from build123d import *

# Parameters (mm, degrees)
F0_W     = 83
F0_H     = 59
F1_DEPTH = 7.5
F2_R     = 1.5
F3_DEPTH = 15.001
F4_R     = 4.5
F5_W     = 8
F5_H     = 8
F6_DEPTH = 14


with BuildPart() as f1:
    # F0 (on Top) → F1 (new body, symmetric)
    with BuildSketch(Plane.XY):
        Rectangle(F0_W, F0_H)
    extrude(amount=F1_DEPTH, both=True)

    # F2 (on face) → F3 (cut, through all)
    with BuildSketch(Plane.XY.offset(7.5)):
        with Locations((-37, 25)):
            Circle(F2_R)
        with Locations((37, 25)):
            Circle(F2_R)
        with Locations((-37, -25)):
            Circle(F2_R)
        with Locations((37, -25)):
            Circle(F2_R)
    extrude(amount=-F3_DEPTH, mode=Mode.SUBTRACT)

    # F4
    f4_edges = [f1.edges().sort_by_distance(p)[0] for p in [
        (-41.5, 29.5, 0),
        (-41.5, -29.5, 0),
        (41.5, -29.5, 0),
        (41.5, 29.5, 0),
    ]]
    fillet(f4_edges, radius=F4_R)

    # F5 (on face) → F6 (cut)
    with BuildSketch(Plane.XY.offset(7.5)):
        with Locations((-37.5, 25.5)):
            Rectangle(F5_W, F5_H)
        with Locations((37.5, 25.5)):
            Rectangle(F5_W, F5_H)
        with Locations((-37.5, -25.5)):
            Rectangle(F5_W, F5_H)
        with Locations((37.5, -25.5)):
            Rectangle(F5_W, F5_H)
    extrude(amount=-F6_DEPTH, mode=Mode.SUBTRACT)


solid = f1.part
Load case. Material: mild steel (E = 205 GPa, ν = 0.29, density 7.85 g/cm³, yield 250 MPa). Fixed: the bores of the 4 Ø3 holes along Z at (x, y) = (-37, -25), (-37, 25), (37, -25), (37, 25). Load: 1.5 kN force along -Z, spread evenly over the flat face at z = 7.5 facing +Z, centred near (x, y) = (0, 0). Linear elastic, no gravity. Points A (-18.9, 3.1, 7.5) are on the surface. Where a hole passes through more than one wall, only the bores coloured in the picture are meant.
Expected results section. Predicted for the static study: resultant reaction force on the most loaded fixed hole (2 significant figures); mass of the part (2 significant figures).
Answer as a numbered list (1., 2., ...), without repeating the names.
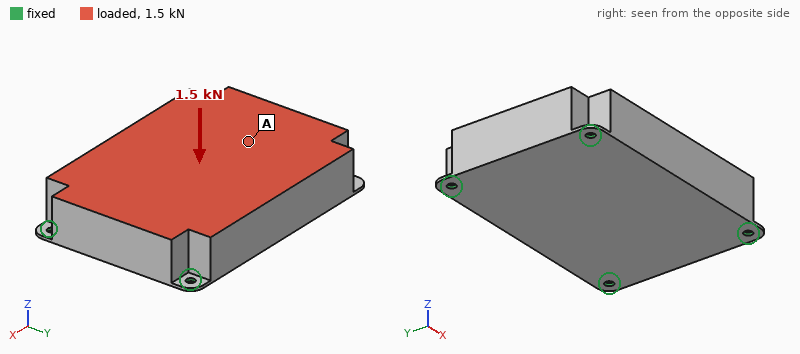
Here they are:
1. 450 N
2. 550 g
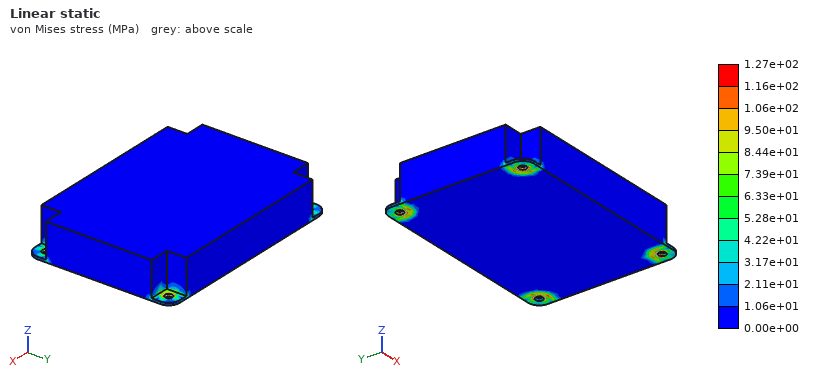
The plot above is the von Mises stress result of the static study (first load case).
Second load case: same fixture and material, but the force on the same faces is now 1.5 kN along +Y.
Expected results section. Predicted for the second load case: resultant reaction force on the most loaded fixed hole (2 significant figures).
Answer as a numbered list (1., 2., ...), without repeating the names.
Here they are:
1. 460 N
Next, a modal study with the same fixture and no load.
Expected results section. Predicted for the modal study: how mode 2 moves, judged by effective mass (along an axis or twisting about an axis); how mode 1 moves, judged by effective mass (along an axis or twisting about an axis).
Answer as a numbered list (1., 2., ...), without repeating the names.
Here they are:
1. along Y
2. along Z
